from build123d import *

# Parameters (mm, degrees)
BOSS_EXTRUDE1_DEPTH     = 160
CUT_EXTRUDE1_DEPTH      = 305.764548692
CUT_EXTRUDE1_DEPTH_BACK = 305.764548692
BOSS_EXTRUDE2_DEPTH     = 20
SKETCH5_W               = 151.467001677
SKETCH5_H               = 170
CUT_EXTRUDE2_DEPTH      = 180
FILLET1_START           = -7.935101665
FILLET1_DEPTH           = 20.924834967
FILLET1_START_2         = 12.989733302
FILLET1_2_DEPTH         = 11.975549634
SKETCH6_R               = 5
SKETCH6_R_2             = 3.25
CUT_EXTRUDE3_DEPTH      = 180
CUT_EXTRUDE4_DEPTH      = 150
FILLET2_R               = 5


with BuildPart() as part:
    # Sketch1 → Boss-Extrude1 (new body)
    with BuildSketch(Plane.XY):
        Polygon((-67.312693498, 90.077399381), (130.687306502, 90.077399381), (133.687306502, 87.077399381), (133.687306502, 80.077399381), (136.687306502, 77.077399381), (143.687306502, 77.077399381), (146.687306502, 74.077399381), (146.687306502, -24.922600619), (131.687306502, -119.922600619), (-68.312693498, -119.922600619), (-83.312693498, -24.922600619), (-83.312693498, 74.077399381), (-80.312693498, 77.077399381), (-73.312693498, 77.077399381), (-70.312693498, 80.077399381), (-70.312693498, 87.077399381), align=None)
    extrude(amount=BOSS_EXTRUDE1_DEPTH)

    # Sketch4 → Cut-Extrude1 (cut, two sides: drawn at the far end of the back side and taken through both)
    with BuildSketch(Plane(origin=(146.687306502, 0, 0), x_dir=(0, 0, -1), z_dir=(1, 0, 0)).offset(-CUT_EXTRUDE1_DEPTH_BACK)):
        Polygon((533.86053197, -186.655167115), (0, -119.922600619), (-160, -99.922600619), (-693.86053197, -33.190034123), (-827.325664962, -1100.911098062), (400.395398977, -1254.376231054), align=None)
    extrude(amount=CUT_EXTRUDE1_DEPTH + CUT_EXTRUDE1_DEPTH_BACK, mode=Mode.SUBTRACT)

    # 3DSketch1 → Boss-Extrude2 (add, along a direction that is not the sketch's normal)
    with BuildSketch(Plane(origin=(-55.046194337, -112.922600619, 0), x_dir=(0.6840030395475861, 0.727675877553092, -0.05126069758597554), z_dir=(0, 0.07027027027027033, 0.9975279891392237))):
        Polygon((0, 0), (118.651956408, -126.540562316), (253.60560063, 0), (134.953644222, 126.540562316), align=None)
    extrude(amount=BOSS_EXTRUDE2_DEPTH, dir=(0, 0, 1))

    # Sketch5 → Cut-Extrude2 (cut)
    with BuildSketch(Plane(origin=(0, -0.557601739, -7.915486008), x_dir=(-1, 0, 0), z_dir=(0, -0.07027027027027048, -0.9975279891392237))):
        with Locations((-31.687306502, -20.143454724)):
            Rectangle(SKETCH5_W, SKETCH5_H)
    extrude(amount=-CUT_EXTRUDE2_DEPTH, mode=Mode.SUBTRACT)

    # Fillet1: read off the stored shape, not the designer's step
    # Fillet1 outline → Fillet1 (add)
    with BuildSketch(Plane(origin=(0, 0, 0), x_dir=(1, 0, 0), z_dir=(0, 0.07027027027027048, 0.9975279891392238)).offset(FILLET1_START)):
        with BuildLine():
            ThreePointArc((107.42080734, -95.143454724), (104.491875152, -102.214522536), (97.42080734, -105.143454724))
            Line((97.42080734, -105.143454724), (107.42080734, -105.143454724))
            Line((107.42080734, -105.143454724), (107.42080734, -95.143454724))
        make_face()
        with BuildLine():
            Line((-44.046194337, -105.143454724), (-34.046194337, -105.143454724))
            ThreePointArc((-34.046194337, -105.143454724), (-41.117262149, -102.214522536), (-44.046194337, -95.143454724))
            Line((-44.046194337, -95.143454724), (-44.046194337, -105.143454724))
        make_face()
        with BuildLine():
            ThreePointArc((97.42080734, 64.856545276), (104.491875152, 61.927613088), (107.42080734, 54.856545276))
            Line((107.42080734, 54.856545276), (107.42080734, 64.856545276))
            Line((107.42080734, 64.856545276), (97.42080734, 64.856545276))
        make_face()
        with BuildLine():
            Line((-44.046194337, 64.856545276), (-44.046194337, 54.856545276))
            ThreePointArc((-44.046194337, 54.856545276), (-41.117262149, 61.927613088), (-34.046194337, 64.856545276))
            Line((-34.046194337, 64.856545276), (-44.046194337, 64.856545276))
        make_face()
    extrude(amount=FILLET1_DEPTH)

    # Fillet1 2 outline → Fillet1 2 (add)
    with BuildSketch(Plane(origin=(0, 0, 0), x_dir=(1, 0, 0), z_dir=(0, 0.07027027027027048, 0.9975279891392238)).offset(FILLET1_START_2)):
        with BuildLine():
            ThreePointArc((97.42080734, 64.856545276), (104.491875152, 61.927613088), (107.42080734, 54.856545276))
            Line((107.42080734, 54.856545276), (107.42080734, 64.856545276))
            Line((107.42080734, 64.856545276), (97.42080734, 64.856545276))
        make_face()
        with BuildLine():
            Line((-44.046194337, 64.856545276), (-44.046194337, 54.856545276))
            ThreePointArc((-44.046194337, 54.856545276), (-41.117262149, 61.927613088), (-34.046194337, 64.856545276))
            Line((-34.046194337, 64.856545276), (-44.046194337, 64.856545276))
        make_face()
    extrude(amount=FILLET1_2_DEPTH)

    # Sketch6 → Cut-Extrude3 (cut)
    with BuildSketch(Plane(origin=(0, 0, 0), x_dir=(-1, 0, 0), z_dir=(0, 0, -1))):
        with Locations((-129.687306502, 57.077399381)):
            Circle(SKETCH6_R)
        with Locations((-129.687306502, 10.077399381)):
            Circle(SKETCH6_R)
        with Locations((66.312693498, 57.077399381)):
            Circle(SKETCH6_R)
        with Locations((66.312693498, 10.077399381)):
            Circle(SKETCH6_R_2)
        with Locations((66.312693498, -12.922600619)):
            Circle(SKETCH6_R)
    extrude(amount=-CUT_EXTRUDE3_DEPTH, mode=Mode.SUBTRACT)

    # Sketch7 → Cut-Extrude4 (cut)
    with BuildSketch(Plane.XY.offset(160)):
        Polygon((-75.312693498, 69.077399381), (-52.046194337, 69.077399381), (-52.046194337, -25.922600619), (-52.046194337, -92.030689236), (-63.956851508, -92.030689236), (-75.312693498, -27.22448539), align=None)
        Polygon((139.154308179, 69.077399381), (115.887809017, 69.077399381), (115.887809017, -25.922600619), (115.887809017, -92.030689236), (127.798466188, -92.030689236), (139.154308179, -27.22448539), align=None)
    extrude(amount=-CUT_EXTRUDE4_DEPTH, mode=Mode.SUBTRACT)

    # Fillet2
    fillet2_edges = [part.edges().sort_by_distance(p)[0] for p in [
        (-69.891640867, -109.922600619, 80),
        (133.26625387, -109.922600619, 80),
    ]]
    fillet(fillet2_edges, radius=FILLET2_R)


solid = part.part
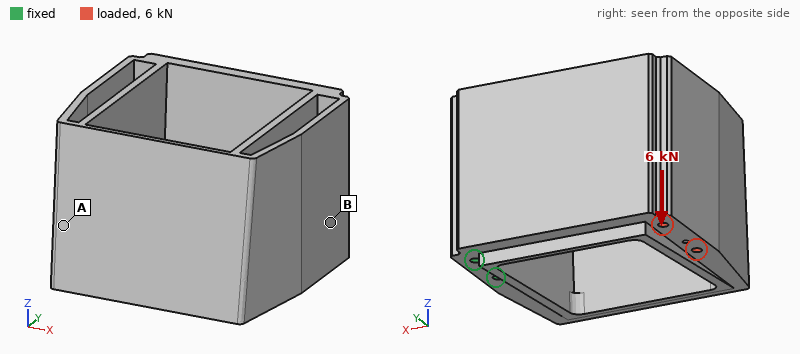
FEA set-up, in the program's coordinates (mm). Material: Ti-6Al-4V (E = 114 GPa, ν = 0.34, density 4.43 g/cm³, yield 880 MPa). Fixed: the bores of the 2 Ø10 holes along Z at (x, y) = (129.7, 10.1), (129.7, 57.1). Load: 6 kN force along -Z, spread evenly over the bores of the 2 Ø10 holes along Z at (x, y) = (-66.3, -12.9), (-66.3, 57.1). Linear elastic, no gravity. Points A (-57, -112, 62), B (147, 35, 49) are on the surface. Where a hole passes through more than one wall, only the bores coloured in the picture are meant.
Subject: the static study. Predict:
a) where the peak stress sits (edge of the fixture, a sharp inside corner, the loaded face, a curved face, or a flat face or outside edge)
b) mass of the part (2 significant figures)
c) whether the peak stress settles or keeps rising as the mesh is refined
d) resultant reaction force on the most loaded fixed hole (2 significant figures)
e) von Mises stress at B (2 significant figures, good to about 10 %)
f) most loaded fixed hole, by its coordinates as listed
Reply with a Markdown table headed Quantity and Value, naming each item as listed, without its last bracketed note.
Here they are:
| Quantity | Value |
|---|---|
| where the peak stress sits | edge of the fixture |
| mass of the part | 8.9 kg |
| whether the peak stress settles or keeps rising as the mesh is refined | keeps rising |
| resultant reaction force on the most loaded fixed hole | 4.2 kN |
| von Mises stress at B | 31 MPa |
| most loaded fixed hole, by its coordinates as listed | (129.7, 10.1) |
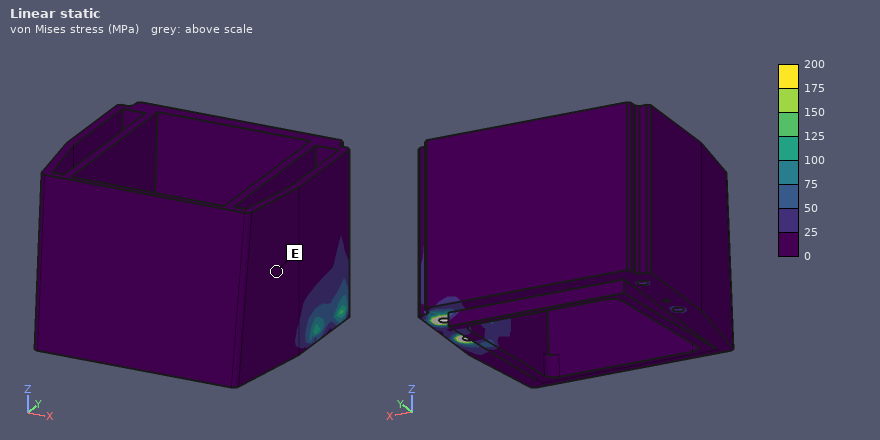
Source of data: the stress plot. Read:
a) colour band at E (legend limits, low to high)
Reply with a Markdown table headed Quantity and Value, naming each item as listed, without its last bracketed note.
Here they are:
| Quantity | Value |
|---|---|
| colour band at E | 0 to 25 MPa |
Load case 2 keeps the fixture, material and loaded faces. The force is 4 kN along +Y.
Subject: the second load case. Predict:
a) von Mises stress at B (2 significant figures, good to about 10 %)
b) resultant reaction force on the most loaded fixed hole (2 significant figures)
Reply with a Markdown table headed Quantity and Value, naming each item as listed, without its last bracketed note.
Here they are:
| Quantity | Value |
|---|---|
| von Mises stress at B | 12 MPa |
| resultant reaction force on the most loaded fixed hole | 13 kN |
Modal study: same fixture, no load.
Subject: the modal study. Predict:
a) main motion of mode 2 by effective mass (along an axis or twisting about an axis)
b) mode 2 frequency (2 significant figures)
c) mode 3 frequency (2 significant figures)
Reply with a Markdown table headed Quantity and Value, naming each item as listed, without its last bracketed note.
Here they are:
| Quantity | Value |
|---|---|
| main motion of mode 2 by effective mass | along Y |
| mode 2 frequency | 230 Hz |
| mode 3 frequency | 420 Hz |
